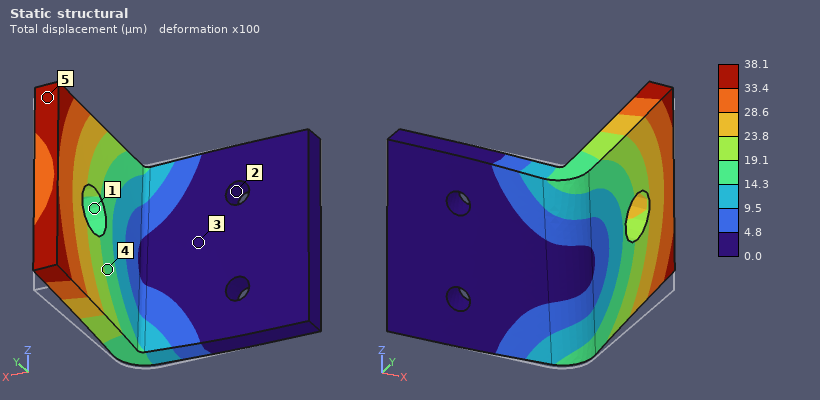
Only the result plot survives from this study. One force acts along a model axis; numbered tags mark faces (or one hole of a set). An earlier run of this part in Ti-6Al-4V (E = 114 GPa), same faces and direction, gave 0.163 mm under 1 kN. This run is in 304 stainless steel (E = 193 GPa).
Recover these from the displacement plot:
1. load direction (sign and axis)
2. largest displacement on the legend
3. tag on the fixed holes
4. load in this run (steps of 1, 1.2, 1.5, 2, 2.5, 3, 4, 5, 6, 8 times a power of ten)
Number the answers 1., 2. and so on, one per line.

1. +Z
2. 38.1 µm
3. 2
4. 400 N
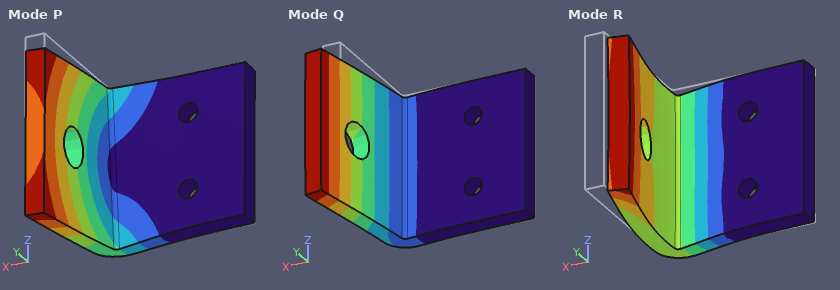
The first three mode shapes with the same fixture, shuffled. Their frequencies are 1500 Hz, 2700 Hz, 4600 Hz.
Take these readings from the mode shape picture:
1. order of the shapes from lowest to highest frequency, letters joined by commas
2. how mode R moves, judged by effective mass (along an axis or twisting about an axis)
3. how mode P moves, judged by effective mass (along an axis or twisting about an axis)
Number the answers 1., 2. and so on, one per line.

1. Q, P, R
2. along Y
3. along Z
